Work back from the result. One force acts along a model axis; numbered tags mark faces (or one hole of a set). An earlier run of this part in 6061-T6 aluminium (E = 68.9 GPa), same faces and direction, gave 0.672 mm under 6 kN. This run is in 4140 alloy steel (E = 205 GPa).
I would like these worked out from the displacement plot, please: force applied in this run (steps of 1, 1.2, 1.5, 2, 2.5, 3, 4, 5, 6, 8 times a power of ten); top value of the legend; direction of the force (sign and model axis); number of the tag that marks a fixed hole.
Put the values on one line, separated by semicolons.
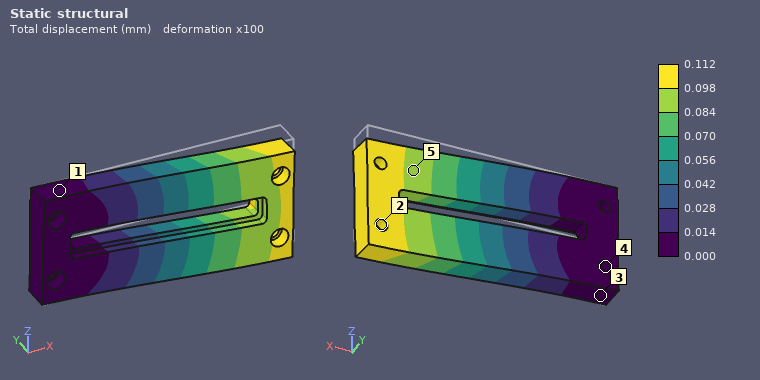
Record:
3 kN; 0.112 mm; -Z; 4
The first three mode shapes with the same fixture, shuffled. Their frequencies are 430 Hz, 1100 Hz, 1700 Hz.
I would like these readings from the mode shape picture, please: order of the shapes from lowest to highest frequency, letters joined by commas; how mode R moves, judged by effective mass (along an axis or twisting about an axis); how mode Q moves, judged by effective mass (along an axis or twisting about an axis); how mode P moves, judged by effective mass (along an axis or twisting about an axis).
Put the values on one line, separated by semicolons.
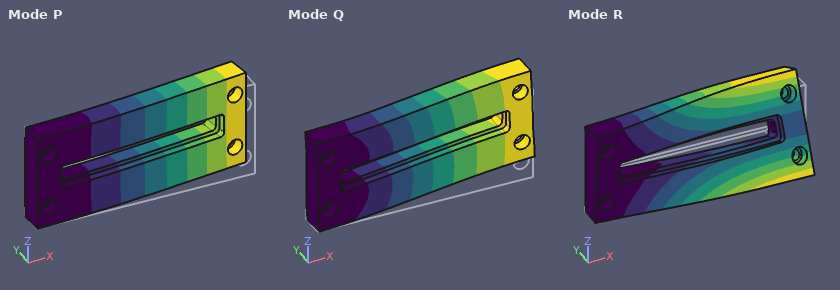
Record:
P, Q, R; twisting about X; along Z; along Y
